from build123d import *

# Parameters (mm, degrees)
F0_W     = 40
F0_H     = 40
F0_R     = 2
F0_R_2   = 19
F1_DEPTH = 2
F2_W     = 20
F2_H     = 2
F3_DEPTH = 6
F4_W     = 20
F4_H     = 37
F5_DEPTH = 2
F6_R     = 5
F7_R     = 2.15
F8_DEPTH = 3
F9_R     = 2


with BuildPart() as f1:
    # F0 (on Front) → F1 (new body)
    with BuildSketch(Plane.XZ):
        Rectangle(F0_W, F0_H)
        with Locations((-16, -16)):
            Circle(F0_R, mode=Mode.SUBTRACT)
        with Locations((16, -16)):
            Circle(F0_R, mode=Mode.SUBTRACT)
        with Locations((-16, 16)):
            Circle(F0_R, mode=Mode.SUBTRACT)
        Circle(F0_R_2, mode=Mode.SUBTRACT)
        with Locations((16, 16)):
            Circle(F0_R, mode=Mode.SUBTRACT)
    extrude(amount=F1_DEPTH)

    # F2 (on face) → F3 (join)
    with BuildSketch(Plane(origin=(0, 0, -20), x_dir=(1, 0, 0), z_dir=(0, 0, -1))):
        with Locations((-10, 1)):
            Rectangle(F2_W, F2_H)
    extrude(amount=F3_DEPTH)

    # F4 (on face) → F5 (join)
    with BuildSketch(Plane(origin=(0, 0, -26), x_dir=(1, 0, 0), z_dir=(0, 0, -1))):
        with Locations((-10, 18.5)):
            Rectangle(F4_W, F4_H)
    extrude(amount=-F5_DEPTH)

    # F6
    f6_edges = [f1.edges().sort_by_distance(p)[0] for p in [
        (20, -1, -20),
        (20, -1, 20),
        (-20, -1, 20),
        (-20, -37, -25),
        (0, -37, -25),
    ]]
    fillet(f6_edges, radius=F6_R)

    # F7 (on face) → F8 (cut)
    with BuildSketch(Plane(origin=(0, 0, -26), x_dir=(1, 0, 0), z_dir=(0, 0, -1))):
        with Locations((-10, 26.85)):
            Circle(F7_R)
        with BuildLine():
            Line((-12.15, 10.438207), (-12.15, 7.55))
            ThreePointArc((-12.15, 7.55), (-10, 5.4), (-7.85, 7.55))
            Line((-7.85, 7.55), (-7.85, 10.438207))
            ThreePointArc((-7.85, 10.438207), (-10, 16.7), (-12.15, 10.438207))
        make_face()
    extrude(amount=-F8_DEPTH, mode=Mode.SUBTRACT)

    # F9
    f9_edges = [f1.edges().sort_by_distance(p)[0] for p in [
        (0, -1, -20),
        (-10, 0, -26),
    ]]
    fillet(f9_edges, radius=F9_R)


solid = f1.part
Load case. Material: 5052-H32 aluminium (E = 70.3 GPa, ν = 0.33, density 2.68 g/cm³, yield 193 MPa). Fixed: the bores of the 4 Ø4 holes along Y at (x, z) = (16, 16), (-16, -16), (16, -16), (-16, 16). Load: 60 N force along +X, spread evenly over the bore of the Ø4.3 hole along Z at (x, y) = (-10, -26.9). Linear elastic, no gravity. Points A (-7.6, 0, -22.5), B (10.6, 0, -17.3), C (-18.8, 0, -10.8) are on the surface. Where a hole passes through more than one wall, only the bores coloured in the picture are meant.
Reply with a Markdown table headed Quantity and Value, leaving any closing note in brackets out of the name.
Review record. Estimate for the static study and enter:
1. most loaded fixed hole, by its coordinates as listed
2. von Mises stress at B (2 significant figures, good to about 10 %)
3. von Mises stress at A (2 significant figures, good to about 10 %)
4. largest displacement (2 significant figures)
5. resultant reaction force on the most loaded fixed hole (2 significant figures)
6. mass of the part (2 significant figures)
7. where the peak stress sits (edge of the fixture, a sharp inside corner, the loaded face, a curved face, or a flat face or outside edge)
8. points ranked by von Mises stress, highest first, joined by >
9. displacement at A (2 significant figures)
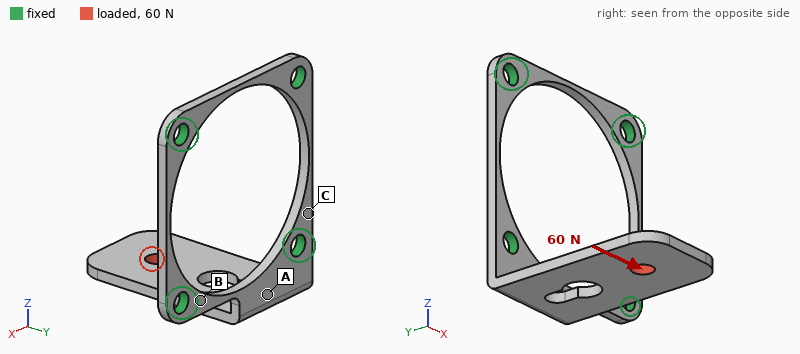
| Quantity | Value |
|---|---|
| most loaded fixed hole, by its coordinates as listed | (-16, -16) |
| von Mises stress at B | 71 MPa |
| von Mises stress at A | 34 MPa |
| largest displacement | 0.32 mm |
| resultant reaction force on the most loaded fixed hole | 52 N |
| mass of the part | 6.1 g |
| where the peak stress sits | a curved face |
| points ranked by von Mises stress, highest first, joined by > | B > A > C |
| displacement at A | 0.048 mm |
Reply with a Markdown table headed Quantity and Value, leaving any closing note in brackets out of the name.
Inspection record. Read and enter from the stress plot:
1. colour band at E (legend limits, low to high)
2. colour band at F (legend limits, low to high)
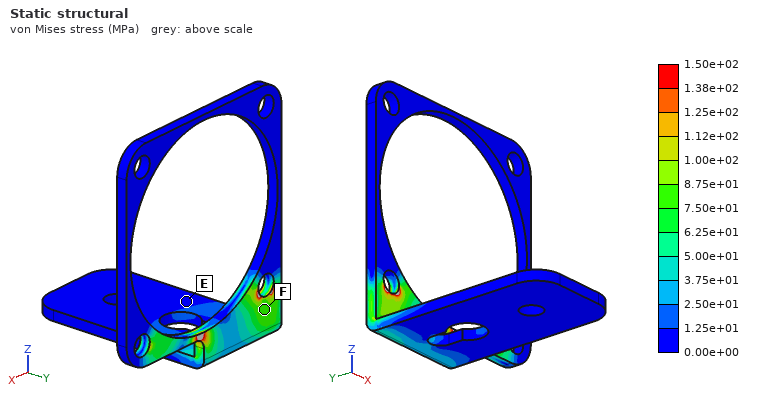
| Quantity | Value |
|---|---|
| colour band at E | 0.00e+00 to 1.25e+01 MPa |
| colour band at F | 7.50e+01 to 8.75e+01 MPa |
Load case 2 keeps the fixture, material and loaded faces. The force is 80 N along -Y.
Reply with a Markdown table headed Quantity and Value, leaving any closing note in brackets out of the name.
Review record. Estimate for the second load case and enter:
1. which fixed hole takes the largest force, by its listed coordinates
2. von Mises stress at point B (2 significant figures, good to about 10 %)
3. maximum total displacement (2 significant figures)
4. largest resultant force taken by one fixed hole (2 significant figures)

| Quantity | Value |
|---|---|
| which fixed hole takes the largest force, by its listed coordinates | (-16, -16) |
| von Mises stress at point B | 23 MPa |
| maximum total displacement | 0.20 mm |
| largest resultant force taken by one fixed hole | 70 N |
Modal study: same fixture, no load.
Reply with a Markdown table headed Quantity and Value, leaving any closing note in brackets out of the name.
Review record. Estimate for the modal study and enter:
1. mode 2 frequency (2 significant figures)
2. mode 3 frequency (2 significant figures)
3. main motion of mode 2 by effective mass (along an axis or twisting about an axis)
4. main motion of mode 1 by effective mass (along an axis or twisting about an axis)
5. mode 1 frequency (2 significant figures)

| Quantity | Value |
|---|---|
| mode 2 frequency | 1700 Hz |
| mode 3 frequency | 4300 Hz |
| main motion of mode 2 by effective mass | along X |
| main motion of mode 1 by effective mass | along Z |
| mode 1 frequency | 850 Hz |
